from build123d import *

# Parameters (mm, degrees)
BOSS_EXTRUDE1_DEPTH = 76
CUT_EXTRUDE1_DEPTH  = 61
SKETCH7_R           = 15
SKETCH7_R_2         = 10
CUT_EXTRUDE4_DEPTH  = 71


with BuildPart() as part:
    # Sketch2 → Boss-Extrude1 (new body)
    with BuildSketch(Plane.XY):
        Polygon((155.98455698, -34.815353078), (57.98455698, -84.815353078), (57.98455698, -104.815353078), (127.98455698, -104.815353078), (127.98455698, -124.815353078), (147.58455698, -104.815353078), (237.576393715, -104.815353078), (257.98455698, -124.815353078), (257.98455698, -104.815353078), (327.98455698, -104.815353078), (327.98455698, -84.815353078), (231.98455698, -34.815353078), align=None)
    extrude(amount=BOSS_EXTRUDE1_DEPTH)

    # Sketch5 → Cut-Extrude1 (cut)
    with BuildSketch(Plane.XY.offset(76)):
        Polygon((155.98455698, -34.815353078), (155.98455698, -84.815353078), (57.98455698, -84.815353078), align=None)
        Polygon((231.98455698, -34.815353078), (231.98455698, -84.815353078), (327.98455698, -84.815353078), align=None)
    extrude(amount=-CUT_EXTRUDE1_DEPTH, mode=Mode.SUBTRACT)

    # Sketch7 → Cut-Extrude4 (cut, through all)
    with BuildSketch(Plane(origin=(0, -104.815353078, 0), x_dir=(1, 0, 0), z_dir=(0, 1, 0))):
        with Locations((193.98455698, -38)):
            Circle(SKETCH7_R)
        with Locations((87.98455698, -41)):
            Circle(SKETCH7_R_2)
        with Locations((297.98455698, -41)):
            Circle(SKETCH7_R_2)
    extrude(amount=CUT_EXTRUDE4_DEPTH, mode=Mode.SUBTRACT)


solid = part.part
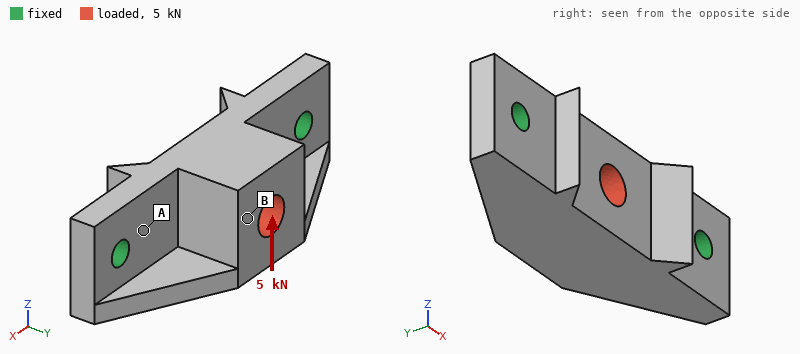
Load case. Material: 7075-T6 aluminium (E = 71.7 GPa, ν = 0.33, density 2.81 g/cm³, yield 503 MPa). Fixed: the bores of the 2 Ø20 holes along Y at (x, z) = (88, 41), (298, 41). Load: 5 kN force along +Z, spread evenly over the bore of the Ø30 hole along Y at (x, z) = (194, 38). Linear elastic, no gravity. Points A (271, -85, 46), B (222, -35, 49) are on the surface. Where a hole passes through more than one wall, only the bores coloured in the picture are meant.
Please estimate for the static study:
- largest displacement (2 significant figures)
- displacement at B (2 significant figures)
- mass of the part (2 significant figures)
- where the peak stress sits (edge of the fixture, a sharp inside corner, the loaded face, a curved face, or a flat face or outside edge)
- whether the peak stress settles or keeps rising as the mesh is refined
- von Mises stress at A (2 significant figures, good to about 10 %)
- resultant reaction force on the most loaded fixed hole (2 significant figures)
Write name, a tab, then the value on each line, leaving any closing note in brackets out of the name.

largest displacement	51 µm
displacement at B	46 µm
mass of the part	2.1 kg
where the peak stress sits	edge of the fixture
whether the peak stress settles or keeps rising as the mesh is refined	keeps rising
von Mises stress at A	11 MPa
resultant reaction force on the most loaded fixed hole	2.5 kN
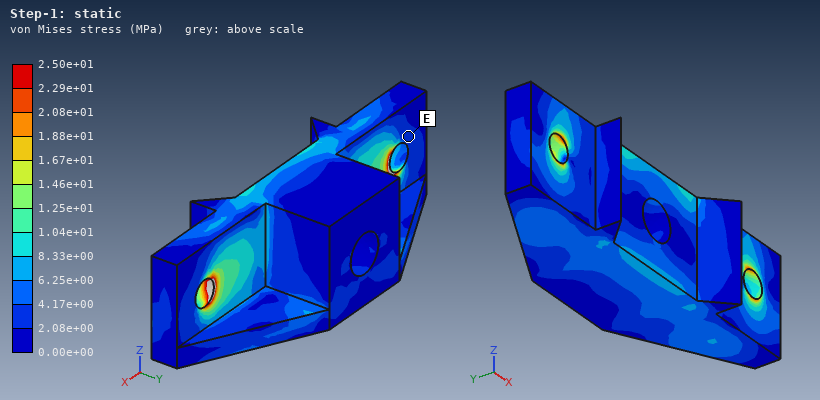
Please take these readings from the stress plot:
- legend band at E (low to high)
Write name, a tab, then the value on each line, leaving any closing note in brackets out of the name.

legend band at E	2.08e+00 to 4.17e+00 MPa
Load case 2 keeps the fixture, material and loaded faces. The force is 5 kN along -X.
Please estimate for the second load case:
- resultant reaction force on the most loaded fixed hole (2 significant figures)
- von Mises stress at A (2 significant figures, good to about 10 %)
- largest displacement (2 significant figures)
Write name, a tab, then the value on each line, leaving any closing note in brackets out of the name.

resultant reaction force on the most loaded fixed hole	2.6 kN
von Mises stress at A	2.5 MPa
largest displacement	6.1 µm
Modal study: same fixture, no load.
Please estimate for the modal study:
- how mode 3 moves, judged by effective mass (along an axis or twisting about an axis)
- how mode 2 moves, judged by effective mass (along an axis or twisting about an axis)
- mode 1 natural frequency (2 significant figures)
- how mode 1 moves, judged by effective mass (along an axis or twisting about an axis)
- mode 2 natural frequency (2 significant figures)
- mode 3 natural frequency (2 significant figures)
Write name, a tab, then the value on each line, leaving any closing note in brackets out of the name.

how mode 3 moves, judged by effective mass	along Z
how mode 2 moves, judged by effective mass	along Y
mode 1 natural frequency	1600 Hz
how mode 1 moves, judged by effective mass	along Z
mode 2 natural frequency	2400 Hz
mode 3 natural frequency	4100 Hz
